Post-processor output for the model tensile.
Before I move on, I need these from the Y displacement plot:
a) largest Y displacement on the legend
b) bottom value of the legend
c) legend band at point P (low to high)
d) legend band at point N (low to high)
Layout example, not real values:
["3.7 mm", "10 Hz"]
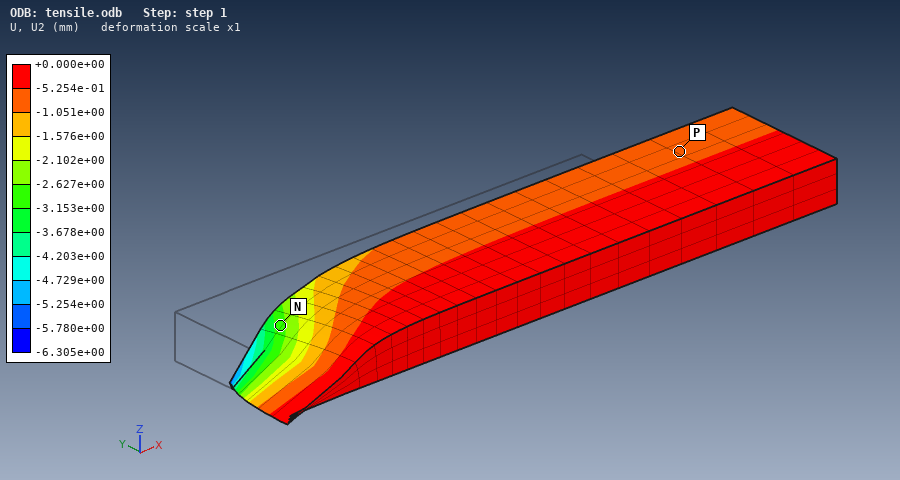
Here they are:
["+0.000e+00 mm", "-6.305e+00 mm", "-1.051e+00 to -5.254e-01 mm", "-3.153e+00 to -2.627e+00 mm"]
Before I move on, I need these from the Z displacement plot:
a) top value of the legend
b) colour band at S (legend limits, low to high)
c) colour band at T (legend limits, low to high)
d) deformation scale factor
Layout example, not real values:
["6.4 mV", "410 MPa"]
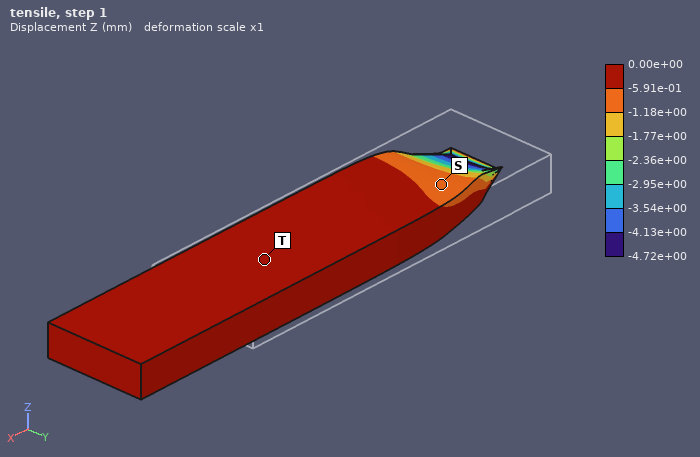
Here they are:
["0.00e+00 mm", "-1.18e+00 to -5.91e-01 mm", "-5.91e-01 to 0.00e+00 mm", "1"]
